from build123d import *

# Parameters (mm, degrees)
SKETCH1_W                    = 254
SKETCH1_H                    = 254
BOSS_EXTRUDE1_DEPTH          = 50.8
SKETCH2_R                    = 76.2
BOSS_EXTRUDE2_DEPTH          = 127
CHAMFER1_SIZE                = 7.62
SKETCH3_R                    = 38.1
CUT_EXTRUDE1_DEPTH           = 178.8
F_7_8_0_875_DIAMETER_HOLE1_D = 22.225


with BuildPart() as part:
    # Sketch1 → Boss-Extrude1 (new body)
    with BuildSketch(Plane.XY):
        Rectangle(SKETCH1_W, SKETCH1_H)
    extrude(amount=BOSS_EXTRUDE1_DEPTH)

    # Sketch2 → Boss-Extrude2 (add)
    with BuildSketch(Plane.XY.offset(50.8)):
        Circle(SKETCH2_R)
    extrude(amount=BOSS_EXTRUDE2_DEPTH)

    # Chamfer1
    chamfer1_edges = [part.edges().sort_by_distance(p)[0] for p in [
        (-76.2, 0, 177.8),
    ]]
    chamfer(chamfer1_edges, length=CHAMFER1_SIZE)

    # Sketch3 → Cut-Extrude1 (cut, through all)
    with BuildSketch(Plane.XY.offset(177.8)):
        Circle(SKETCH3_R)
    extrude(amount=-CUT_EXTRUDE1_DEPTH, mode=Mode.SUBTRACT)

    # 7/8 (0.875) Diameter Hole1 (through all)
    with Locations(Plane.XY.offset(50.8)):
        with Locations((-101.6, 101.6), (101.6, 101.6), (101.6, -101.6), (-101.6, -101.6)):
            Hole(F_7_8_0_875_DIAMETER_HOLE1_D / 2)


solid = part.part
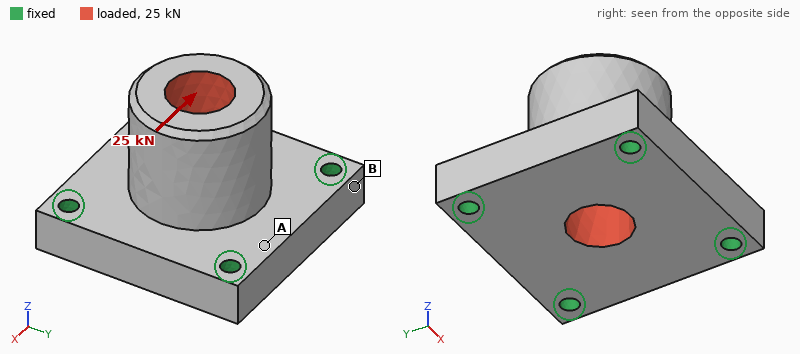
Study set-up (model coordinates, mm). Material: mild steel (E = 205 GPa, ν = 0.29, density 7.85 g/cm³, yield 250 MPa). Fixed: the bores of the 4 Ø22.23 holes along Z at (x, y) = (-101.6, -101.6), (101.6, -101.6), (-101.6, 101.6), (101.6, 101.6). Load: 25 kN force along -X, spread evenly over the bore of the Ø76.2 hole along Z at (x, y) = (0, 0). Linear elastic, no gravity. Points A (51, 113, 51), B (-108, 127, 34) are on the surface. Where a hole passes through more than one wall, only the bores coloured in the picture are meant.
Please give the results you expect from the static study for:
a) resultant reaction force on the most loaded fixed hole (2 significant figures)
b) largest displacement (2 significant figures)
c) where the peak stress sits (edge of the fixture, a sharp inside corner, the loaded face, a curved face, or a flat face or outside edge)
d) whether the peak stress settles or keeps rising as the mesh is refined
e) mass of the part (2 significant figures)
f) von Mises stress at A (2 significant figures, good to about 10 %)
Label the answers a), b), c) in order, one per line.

a) 8.1 kN
b) 8.1 µm
c) edge of the fixture
d) keeps rising
e) 37 kg
f) 2.1 MPa
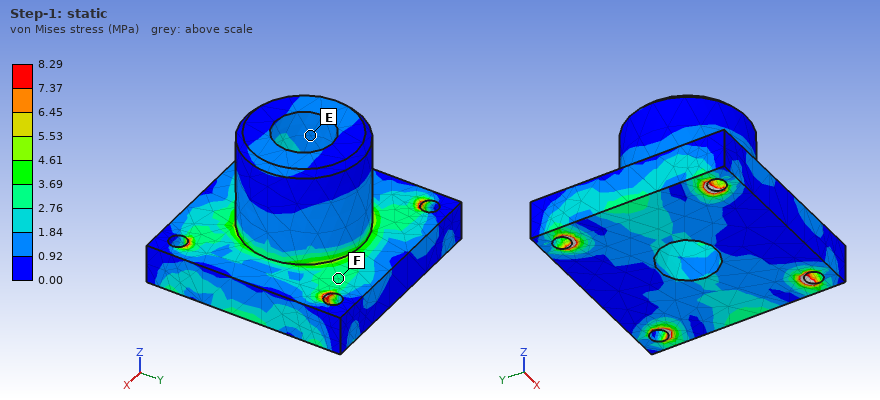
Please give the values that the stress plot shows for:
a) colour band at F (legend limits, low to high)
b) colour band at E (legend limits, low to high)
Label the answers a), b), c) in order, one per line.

a) 2.76 to 3.69 MPa
b) 0.92 to 1.84 MPa
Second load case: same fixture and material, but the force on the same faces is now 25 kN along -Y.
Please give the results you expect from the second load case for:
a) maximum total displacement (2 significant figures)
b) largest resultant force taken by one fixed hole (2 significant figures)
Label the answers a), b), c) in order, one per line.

a) 8.1 µm
b) 8.1 kN
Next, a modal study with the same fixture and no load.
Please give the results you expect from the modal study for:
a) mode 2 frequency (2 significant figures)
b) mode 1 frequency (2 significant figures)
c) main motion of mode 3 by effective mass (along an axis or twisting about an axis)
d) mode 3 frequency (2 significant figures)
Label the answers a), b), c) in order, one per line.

a) 2300 Hz
b) 2300 Hz
c) along Z
d) 2700 Hz
